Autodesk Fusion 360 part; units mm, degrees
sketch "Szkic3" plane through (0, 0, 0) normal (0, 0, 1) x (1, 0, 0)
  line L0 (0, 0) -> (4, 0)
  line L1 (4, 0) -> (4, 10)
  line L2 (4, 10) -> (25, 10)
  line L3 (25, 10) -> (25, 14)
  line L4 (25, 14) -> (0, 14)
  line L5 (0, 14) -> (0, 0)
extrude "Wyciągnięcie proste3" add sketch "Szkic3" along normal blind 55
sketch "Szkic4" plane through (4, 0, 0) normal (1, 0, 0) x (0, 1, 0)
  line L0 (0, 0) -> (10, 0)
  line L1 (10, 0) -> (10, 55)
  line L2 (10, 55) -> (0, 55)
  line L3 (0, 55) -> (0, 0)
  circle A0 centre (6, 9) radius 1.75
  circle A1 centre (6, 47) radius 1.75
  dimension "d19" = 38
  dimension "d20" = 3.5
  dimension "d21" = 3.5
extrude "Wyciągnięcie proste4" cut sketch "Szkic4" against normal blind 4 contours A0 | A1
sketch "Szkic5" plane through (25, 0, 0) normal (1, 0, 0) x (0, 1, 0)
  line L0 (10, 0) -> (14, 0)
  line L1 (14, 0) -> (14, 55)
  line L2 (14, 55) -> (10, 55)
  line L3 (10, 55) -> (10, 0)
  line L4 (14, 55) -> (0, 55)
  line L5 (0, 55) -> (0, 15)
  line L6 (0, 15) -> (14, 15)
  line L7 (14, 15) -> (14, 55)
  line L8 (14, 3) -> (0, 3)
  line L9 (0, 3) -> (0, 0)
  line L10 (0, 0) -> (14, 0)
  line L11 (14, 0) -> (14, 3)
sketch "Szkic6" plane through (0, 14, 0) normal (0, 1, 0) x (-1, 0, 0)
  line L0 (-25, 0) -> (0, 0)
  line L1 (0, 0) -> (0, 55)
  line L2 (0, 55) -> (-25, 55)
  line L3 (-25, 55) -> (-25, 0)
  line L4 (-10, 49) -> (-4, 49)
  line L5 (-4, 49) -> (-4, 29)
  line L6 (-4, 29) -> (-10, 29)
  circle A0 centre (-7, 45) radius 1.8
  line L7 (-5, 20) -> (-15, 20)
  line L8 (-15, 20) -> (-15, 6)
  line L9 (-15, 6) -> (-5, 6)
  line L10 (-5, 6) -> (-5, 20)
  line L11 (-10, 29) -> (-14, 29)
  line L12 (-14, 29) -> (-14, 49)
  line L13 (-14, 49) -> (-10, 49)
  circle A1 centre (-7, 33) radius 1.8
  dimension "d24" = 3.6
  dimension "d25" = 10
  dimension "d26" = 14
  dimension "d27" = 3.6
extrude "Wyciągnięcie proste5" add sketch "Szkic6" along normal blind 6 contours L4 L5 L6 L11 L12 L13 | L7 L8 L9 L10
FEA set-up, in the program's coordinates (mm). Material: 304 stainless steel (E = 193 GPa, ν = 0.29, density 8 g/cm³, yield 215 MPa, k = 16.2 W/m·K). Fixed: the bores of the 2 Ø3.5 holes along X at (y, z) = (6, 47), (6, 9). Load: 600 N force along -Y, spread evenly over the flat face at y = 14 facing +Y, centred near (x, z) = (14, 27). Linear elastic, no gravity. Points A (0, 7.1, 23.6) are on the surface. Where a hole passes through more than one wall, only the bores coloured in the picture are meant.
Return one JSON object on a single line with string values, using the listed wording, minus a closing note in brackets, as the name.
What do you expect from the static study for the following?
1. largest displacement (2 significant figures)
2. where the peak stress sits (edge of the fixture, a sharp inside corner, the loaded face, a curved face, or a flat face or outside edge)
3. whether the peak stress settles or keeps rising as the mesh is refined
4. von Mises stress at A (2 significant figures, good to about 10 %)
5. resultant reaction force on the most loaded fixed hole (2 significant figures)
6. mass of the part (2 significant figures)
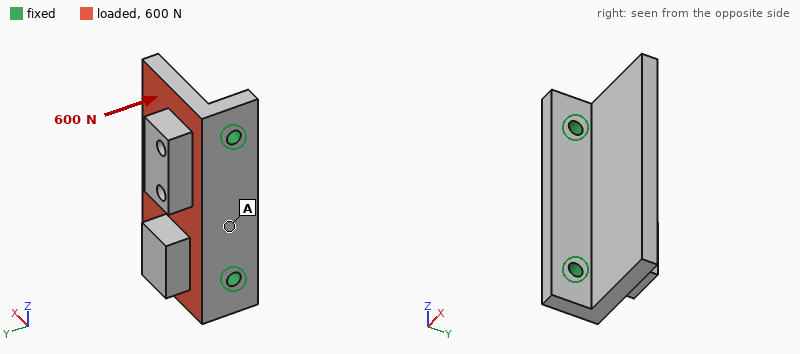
{"largest displacement": "35 µm", "where the peak stress sits": "edge of the fixture", "whether the peak stress settles or keeps rising as the mesh is refined": "keeps rising", "von Mises stress at A": "18 MPa", "resultant reaction force on the most loaded fixed hole": "320 N", "mass of the part": "76 g"}
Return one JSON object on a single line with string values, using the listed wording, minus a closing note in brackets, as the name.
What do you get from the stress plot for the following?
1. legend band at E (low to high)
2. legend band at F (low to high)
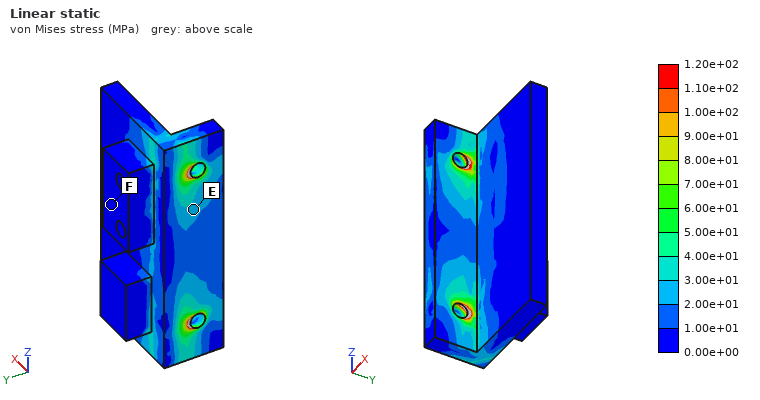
{"legend band at E": "2.00e+01 to 3.00e+01 MPa", "legend band at F": "0.00e+00 to 1.00e+01 MPa"}
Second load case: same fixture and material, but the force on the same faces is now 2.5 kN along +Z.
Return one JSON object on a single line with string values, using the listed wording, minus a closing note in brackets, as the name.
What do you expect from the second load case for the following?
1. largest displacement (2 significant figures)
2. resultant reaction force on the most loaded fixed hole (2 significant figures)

{"largest displacement": "8.8 µm", "resultant reaction force on the most loaded fixed hole": "1.5 kN"}
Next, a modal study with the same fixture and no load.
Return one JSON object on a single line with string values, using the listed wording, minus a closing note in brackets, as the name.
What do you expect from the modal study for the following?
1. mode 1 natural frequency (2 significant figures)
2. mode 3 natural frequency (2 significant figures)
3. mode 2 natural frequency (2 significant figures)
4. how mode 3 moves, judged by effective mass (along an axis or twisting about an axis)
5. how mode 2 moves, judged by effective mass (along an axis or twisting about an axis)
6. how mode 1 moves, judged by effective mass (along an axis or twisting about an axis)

{"mode 1 natural frequency": "3600 Hz", "mode 3 natural frequency": "13 kHz", "mode 2 natural frequency": "7400 Hz", "how mode 3 moves, judged by effective mass": "along X", "how mode 2 moves, judged by effective mass": "twisting about X", "how mode 1 moves, judged by effective mass": "along Y"}
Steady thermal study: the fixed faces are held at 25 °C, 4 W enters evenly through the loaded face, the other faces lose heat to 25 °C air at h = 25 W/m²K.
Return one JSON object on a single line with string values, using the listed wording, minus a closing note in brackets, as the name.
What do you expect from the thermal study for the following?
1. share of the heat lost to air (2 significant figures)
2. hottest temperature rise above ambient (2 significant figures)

{"share of the heat lost to air": "27 %", "hottest temperature rise above ambient": "17 K"}
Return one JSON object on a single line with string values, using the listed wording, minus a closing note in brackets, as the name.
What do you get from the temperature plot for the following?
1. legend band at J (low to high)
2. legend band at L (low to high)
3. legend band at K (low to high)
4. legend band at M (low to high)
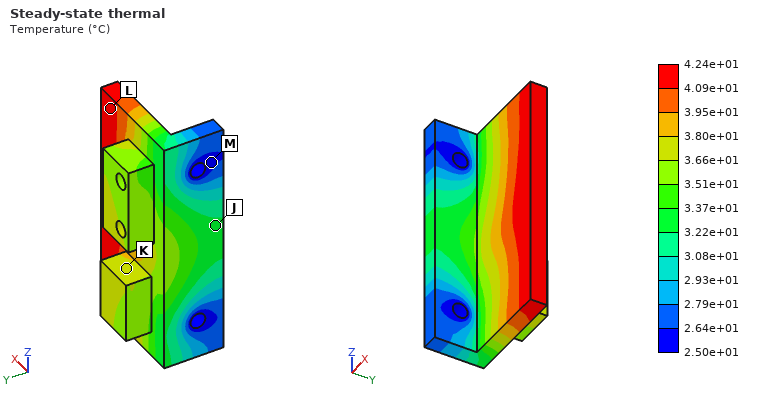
{"legend band at J": "3.22e+01 to 3.37e+01 °C", "legend band at L": "4.09e+01 to 4.24e+01 °C", "legend band at K": "3.66e+01 to 3.80e+01 °C", "legend band at M": "2.50e+01 to 2.64e+01 °C"}
